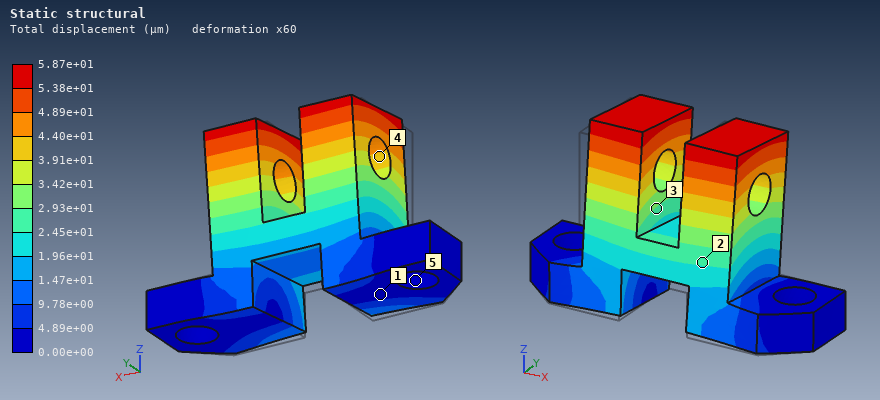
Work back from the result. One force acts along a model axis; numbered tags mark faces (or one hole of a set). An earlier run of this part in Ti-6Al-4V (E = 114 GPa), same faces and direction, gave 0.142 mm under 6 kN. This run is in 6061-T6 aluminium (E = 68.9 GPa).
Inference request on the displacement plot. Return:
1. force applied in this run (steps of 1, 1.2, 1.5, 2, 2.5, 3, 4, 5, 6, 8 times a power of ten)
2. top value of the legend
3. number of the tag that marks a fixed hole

1.5 kN
5.87e+01 µm
5
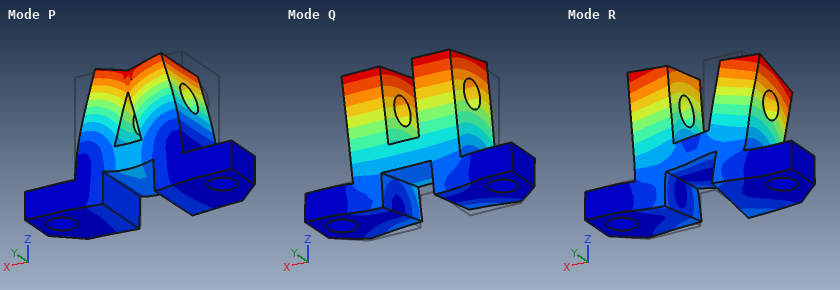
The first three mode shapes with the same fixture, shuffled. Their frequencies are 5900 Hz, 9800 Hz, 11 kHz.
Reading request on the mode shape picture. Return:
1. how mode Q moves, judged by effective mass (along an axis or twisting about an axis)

along Y
